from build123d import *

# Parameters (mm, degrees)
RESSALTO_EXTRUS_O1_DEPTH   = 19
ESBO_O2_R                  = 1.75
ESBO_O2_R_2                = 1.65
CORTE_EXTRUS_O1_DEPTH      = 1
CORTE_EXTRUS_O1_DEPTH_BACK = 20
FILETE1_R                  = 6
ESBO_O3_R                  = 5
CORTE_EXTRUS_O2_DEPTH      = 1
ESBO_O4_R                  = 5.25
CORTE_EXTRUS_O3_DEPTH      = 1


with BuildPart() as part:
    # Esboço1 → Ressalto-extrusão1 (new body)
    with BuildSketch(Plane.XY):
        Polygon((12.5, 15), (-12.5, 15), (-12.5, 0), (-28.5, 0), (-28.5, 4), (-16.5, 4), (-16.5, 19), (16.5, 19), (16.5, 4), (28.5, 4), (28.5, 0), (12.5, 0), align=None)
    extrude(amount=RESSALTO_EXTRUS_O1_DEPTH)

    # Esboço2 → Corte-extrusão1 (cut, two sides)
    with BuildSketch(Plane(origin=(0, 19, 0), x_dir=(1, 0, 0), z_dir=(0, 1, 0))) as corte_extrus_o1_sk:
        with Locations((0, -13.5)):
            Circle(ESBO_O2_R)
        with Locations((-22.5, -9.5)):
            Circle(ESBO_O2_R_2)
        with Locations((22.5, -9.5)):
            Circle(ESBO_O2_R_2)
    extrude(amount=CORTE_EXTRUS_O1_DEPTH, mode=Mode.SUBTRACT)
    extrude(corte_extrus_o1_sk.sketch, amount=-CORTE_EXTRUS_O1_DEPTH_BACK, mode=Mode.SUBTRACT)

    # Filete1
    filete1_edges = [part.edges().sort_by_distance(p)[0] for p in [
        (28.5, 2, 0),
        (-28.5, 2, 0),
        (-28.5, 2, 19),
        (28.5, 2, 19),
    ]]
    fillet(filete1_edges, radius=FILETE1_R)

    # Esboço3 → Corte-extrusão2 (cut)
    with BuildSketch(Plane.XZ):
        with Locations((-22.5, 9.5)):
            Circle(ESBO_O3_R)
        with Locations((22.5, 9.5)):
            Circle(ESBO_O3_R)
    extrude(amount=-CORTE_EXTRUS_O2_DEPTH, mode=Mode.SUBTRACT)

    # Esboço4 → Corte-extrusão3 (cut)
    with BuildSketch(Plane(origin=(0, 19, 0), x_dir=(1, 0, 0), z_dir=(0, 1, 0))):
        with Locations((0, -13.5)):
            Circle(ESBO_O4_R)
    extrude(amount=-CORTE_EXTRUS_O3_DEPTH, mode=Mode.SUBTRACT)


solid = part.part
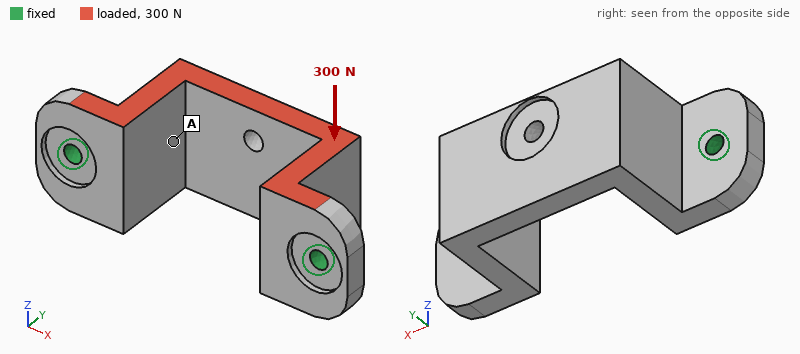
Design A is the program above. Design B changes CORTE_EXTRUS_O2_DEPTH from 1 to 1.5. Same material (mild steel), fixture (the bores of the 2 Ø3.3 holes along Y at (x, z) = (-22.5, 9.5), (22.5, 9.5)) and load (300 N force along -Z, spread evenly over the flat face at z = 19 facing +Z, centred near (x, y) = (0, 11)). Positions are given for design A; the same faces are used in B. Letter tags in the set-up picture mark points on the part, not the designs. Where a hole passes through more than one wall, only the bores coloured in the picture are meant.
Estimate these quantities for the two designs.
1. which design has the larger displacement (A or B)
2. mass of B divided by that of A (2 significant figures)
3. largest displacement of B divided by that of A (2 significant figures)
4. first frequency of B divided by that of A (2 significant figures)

B
0.99
1.2
0.89
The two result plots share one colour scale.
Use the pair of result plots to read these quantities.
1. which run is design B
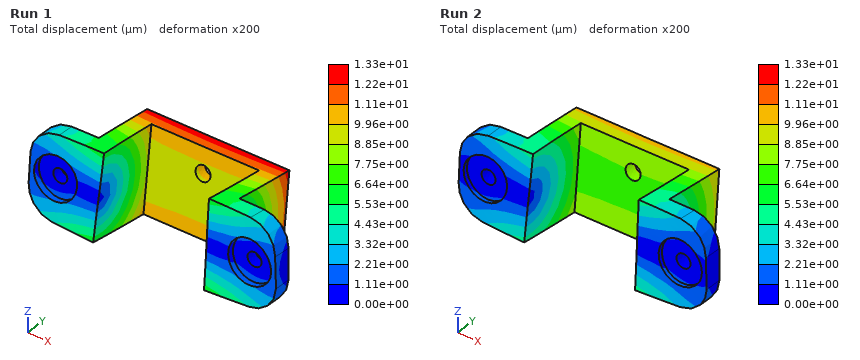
Run 1
